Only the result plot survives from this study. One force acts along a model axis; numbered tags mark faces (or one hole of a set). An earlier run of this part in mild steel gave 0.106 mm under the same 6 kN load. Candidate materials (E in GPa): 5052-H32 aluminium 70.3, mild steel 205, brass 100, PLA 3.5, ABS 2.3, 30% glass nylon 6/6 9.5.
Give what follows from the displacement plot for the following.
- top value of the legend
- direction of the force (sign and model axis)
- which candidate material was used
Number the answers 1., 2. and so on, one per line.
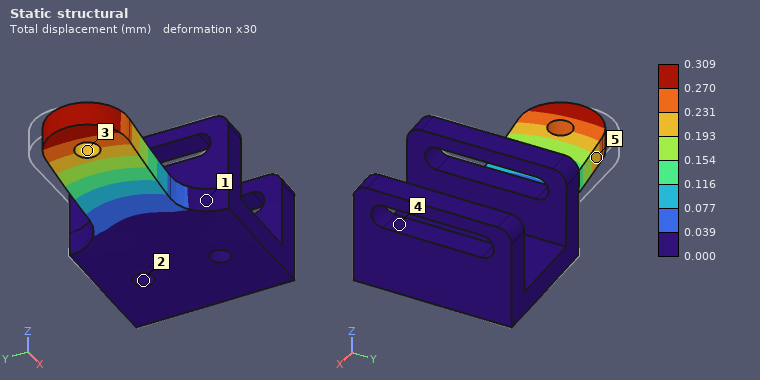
1. 0.309 mm
2. -Y
3. 5052-H32 aluminium
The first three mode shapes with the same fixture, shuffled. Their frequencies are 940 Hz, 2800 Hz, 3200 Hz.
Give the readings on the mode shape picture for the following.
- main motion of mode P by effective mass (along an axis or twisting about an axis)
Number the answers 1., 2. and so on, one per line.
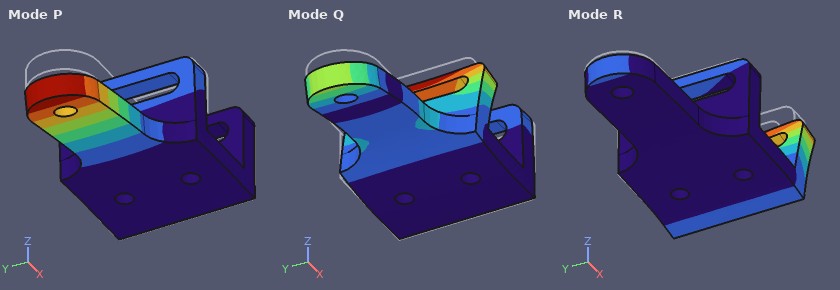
1. along Z
